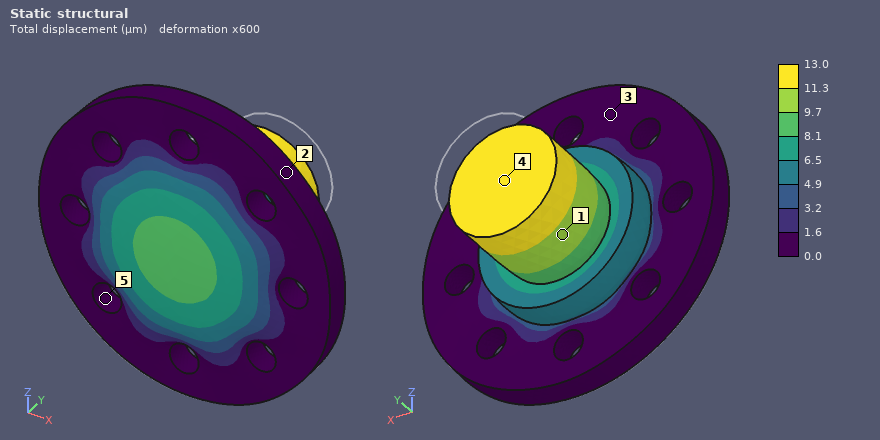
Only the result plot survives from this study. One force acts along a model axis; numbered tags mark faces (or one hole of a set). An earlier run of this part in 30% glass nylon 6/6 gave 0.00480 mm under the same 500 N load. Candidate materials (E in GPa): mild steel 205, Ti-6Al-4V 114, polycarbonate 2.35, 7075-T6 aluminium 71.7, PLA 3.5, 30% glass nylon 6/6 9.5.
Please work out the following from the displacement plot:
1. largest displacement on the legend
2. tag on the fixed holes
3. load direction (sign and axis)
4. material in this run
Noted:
13.0 µm
5
-Y
PLA
